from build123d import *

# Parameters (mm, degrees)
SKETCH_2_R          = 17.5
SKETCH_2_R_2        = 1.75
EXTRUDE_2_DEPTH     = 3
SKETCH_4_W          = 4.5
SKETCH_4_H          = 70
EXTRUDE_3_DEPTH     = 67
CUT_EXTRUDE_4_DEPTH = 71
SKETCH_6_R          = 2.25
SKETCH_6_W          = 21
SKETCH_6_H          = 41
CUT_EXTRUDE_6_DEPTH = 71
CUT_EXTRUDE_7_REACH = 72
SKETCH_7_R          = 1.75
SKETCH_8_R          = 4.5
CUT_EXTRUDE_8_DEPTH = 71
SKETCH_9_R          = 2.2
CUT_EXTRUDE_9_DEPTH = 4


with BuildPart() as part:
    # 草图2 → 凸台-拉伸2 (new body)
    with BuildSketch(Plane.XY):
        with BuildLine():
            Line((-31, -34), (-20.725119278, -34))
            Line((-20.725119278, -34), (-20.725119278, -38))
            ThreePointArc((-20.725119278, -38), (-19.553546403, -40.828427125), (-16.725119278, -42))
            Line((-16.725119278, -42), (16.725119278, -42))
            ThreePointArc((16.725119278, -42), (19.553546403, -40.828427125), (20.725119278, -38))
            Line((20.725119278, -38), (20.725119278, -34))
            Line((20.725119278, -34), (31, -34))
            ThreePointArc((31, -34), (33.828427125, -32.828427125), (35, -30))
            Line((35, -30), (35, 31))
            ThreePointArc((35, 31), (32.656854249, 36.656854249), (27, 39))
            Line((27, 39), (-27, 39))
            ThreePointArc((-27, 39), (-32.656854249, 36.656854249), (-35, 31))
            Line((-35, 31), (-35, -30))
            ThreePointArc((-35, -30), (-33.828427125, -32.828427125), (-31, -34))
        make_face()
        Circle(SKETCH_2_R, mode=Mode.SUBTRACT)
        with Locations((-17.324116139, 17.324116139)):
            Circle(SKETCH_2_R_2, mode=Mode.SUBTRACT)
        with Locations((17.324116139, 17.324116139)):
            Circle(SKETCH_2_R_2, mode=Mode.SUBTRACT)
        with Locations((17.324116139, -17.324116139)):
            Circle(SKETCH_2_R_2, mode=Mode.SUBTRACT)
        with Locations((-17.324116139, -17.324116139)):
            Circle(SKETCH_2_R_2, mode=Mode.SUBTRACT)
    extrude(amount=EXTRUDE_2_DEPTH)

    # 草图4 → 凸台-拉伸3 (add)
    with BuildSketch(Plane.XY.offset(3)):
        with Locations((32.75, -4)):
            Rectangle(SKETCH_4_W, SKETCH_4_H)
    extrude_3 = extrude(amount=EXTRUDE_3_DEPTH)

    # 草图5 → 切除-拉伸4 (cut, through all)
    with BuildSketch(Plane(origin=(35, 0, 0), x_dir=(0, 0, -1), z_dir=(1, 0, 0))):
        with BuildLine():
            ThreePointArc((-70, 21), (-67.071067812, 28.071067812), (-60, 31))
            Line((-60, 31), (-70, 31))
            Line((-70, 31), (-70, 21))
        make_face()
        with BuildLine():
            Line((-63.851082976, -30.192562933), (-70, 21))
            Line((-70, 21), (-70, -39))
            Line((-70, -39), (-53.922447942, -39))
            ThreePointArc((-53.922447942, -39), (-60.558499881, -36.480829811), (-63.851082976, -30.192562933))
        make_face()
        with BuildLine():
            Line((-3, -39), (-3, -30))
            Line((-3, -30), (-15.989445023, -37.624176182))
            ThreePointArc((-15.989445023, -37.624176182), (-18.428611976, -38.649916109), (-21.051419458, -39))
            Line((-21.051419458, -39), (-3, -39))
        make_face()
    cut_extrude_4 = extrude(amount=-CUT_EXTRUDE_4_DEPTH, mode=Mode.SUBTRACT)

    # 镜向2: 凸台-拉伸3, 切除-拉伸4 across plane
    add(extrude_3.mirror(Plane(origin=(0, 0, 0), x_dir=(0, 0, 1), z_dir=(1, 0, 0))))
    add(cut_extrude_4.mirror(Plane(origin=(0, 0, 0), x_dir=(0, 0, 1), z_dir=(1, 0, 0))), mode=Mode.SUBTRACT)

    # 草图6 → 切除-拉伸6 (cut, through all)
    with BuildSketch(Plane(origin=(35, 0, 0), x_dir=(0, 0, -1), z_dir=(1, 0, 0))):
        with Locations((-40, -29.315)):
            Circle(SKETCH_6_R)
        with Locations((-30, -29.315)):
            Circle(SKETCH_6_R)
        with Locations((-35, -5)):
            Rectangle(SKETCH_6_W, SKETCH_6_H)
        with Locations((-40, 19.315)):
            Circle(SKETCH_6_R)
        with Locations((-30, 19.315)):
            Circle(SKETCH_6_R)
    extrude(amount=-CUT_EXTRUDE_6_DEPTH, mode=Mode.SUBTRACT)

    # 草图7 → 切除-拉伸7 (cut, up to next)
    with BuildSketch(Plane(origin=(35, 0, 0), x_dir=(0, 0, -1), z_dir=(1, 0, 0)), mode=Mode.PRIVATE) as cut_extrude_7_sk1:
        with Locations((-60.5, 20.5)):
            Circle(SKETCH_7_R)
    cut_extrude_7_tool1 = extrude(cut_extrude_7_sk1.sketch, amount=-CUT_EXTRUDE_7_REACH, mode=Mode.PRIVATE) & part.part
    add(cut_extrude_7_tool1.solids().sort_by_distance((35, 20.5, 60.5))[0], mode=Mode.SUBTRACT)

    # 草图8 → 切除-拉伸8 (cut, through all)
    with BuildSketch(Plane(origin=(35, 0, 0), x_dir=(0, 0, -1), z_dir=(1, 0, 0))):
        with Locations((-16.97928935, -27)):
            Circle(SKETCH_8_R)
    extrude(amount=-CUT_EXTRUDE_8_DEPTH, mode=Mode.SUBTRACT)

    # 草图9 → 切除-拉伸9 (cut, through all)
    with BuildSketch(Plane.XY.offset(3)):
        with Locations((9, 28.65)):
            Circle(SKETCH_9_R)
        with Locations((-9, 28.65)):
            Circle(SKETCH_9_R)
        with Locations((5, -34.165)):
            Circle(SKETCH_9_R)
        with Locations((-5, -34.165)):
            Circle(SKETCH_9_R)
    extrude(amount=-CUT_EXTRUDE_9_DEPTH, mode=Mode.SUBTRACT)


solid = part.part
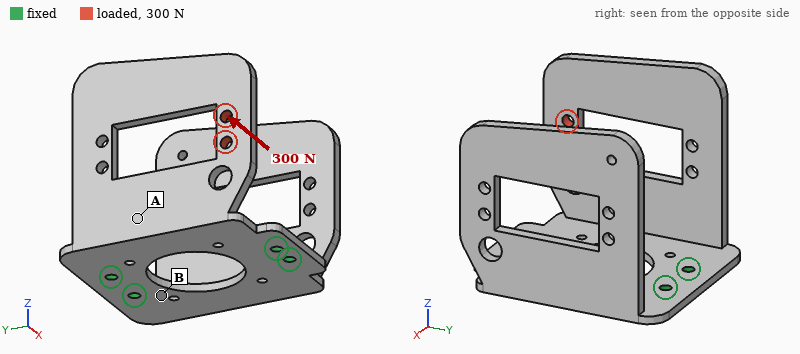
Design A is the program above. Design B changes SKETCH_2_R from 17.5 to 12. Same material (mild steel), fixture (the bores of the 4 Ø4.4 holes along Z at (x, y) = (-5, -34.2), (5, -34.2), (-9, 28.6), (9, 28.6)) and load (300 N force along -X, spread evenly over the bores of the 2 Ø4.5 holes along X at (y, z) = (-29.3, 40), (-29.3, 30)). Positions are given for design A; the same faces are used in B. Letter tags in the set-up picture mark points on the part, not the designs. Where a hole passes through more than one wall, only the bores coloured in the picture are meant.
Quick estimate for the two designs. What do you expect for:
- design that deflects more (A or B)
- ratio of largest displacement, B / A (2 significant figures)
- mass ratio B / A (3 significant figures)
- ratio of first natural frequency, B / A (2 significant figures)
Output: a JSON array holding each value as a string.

["A", "0.90", "1.04", "1.1"]
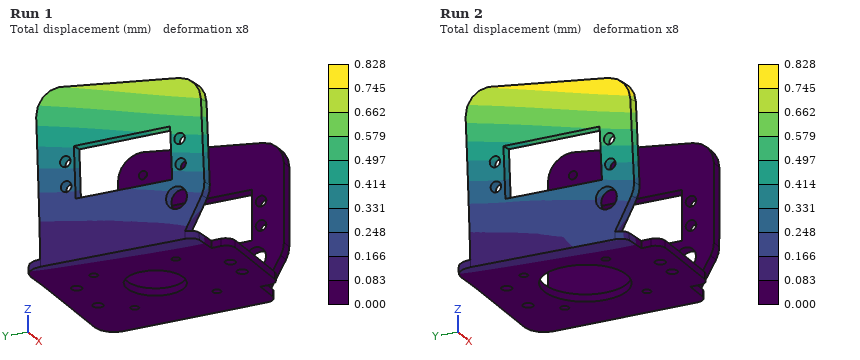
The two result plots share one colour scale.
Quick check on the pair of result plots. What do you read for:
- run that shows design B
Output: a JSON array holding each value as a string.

["Run 1"]
